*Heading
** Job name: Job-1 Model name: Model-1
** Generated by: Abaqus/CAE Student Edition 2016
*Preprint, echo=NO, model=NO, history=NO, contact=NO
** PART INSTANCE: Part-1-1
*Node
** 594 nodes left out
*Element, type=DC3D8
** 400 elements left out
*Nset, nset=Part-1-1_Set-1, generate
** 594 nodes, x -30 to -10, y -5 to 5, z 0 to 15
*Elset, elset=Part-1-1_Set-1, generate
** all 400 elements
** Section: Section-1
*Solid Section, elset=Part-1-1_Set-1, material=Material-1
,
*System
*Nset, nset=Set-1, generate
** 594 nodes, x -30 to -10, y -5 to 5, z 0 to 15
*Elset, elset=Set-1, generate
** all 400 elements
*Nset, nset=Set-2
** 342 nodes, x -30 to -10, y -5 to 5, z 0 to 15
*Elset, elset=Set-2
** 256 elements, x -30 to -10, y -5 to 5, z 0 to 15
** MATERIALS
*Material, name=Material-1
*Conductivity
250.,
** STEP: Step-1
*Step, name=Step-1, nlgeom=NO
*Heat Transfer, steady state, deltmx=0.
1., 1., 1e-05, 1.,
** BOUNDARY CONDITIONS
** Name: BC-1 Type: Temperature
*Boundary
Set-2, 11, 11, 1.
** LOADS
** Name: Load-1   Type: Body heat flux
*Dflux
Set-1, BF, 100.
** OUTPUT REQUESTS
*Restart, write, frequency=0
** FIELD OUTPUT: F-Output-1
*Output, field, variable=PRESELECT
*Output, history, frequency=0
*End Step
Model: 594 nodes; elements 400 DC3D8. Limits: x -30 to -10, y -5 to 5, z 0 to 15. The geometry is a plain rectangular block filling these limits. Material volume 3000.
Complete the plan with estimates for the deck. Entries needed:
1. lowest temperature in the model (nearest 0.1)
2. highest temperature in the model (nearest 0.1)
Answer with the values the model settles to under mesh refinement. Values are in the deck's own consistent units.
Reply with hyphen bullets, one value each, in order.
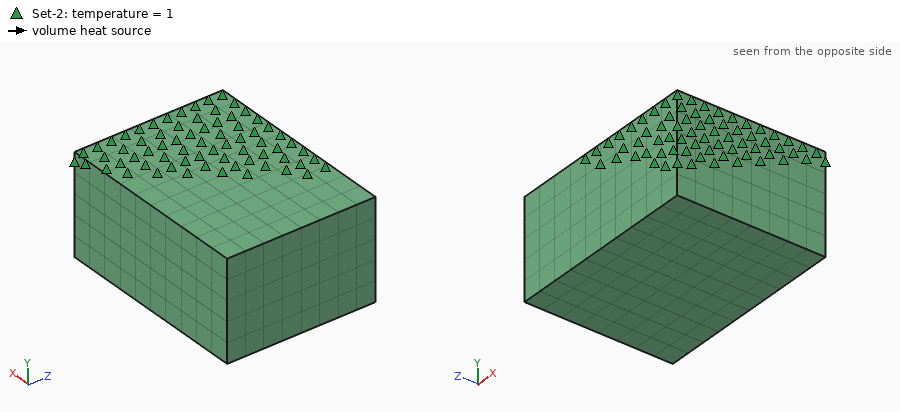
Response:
- 1.0
- 4.8
